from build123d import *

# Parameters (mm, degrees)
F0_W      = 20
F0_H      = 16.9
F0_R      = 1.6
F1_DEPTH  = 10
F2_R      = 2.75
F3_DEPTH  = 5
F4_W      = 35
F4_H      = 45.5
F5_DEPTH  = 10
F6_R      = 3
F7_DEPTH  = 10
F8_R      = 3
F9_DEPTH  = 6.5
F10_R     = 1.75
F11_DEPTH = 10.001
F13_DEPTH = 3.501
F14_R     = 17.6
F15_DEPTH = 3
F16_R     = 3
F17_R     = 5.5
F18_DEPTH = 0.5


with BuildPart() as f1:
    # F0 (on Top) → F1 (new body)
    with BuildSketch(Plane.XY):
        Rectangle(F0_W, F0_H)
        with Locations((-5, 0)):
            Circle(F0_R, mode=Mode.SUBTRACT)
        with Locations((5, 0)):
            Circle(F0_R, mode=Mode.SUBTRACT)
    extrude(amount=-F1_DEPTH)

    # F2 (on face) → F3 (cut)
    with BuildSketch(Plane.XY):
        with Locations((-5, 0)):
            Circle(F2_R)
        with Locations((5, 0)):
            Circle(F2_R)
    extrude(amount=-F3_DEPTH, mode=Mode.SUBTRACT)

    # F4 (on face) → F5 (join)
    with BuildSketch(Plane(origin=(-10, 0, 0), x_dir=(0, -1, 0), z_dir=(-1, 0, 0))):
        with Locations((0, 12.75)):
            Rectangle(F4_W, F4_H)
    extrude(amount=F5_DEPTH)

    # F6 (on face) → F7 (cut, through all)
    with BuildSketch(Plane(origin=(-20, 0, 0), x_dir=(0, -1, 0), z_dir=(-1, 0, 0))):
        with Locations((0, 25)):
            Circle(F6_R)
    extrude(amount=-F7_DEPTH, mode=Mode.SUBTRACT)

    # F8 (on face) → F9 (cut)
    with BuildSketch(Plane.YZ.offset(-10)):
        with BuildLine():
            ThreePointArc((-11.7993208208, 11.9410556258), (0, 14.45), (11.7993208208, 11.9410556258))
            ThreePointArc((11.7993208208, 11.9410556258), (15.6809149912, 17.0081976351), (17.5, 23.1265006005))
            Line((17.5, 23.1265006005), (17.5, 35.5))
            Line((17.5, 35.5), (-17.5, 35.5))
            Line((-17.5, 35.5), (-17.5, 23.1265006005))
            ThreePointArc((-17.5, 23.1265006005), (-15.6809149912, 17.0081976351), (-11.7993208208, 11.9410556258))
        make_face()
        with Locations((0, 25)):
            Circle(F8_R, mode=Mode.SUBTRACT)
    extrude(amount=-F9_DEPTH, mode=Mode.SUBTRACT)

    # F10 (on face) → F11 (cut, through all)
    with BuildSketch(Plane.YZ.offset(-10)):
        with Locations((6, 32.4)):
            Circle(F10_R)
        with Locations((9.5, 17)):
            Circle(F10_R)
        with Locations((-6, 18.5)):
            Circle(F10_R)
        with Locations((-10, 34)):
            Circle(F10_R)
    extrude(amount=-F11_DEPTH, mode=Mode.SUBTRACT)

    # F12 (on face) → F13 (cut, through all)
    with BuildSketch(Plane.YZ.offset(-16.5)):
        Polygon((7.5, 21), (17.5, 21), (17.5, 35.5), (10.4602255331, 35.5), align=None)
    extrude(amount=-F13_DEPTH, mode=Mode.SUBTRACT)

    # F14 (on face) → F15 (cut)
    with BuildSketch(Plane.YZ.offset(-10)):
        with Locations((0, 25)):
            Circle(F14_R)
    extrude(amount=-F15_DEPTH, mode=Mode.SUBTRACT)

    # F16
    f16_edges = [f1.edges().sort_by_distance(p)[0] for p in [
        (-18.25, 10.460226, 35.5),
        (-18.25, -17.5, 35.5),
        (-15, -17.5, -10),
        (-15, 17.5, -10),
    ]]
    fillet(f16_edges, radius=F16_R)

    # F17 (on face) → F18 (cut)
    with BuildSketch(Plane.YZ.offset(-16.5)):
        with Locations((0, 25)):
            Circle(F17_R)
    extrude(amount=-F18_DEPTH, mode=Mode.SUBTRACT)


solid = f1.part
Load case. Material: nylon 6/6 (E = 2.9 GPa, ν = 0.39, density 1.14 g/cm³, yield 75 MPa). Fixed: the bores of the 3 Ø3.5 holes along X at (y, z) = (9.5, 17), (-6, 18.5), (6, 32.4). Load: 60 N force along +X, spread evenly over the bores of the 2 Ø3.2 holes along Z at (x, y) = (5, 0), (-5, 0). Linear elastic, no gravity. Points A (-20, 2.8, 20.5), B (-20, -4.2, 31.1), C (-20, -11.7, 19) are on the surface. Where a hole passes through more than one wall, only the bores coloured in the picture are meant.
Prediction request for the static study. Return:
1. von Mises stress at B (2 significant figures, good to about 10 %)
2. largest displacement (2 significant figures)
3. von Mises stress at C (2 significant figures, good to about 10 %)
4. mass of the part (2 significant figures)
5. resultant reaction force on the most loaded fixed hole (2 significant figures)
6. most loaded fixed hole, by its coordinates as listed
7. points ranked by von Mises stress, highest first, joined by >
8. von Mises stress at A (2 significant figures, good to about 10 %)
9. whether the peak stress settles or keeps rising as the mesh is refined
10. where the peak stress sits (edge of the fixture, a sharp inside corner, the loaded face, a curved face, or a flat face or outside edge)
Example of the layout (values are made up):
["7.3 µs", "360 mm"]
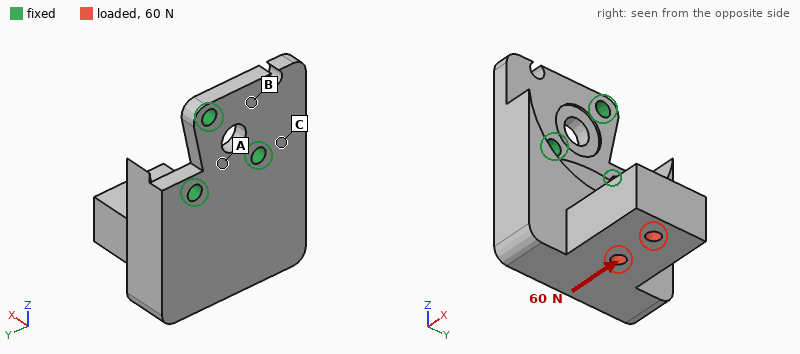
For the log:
["2.2 MPa", "0.72 mm", "7.5 MPa", "15 g", "40 N", "(9.5, 17)", "C > A > B", "4.3 MPa", "keeps rising", "edge of the fixture"]
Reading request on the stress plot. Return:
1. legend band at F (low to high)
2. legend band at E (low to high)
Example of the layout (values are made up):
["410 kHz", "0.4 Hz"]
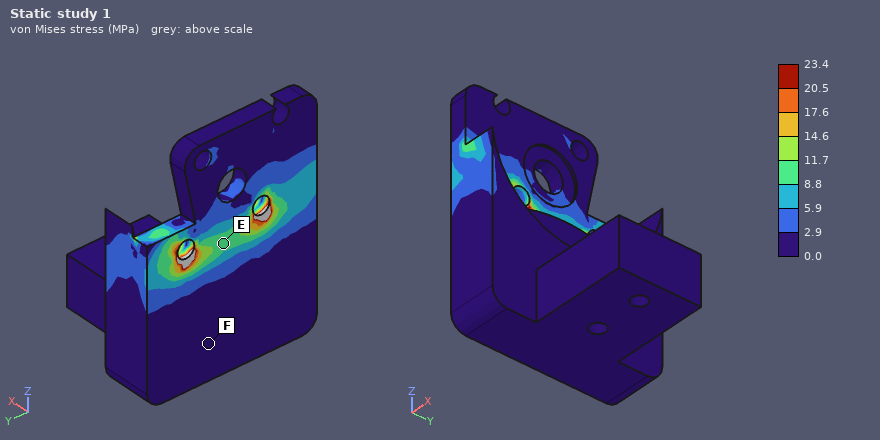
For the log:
["0.0 to 2.9 MPa", "8.8 to 11.7 MPa"]
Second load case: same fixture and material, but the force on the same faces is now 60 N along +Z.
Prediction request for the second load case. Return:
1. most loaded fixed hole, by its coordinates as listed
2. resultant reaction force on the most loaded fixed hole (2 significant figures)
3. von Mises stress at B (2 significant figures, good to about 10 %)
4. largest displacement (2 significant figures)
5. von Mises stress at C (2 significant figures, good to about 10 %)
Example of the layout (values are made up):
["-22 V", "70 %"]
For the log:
["(-6, 18.5)", "34 N", "1.9 MPa", "0.61 mm", "5.5 MPa"]
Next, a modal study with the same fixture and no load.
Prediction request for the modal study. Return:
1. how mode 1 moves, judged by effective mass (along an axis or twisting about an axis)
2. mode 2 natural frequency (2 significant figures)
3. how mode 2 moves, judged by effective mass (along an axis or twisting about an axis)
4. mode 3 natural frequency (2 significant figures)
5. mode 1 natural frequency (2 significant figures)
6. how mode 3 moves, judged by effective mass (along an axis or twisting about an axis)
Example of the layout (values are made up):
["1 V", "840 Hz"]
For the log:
["along X", "1800 Hz", "along Y", "3000 Hz", "610 Hz", "along Y"]
